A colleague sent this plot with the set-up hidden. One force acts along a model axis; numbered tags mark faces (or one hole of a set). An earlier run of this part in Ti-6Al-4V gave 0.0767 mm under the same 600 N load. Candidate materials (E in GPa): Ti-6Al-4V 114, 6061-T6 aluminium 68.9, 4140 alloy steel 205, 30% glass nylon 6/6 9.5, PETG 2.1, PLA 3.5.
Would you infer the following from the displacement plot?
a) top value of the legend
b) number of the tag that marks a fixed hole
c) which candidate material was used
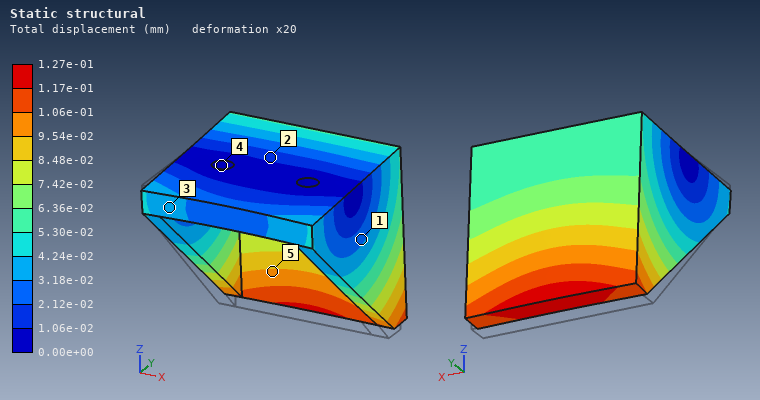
1.27e-01 mm
4
6061-T6 aluminium
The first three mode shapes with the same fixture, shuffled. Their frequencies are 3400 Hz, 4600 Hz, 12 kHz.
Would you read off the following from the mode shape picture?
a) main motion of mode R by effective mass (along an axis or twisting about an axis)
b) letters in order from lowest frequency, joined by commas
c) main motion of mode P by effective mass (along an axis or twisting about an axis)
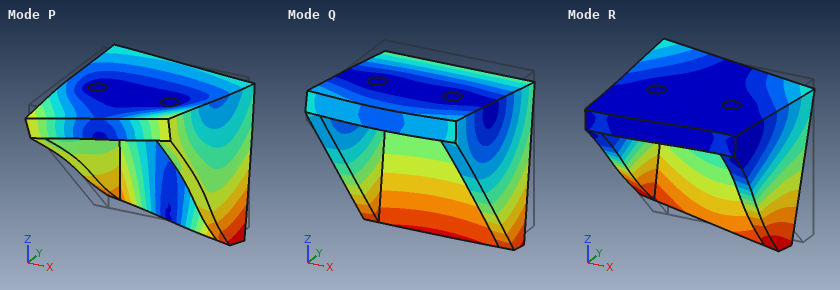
along X
Q, R, P
along X
